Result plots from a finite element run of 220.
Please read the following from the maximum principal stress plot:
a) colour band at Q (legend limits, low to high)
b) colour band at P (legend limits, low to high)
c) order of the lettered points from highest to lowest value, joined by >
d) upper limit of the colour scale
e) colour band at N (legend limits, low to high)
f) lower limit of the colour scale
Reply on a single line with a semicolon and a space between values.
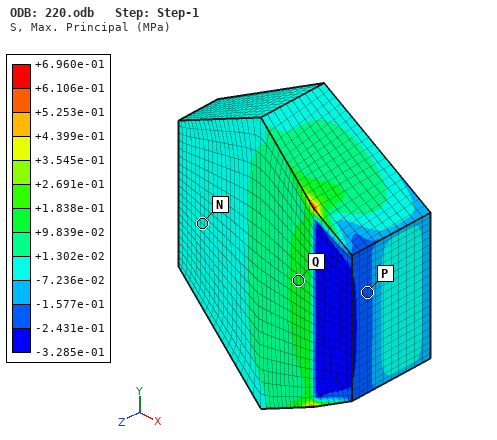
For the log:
+9.839e-02 to +1.838e-01 MPa; -2.431e-01 to -1.577e-01 MPa; Q > N > P; +6.960e-01 MPa; -7.236e-02 to +1.302e-02 MPa; -3.285e-01 MPa
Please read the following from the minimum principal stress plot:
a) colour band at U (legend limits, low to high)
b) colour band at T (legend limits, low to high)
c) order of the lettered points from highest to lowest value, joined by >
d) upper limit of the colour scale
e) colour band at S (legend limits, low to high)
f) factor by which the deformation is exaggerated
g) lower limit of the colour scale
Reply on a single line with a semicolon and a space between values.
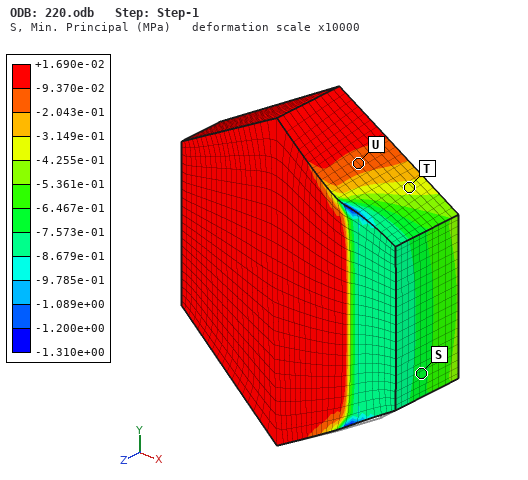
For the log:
-2.043e-01 to -9.370e-02 MPa; -4.255e-01 to -3.149e-01 MPa; U > T > S; +1.690e-02 MPa; -7.573e-01 to -6.467e-01 MPa; 10000; -1.310e+00 MPa
